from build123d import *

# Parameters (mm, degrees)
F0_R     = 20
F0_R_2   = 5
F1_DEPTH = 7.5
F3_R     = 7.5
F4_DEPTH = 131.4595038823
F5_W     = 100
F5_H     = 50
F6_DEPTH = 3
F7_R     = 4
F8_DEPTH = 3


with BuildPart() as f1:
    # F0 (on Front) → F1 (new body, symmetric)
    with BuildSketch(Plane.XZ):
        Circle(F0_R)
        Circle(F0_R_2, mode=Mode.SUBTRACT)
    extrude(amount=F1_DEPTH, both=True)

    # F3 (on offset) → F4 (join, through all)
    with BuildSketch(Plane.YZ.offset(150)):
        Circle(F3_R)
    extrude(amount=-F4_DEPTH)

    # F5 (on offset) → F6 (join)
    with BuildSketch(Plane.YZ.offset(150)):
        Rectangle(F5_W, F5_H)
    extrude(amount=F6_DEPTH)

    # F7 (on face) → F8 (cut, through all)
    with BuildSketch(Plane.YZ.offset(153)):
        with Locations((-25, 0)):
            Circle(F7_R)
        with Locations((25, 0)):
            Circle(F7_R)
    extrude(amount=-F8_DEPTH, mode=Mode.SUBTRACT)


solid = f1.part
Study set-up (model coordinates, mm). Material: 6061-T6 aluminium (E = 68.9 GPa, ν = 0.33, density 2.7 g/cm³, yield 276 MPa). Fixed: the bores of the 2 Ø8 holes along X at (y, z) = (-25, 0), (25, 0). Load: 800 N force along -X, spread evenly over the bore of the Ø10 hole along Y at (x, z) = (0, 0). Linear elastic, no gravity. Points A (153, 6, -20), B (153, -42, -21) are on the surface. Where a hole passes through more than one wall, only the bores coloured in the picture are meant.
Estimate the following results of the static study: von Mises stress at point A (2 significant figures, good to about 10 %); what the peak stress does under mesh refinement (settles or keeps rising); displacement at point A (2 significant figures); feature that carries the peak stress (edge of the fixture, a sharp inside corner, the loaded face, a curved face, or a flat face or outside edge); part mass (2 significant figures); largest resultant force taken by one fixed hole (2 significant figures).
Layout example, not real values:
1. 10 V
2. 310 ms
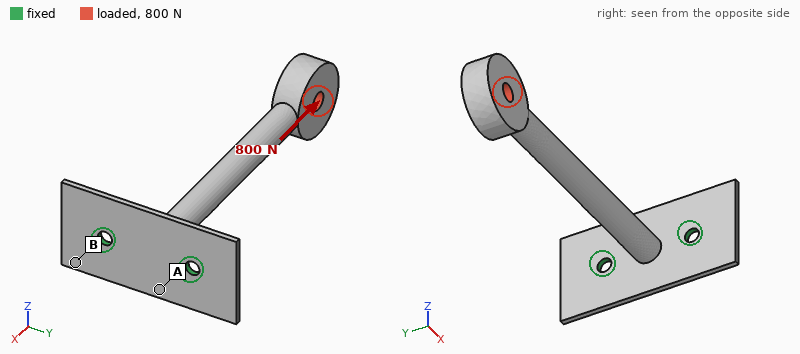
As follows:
1. 17 MPa
2. keeps rising
3. 40 µm
4. edge of the fixture
5. 150 g
6. 410 N
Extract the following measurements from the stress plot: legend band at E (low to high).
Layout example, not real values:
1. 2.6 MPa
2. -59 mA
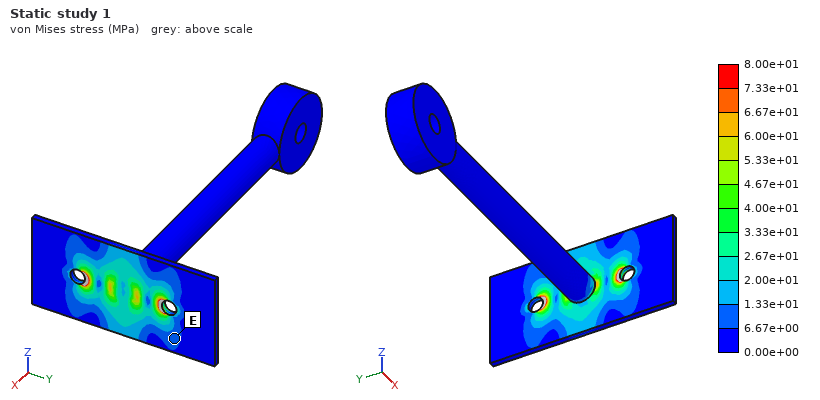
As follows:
1. 6.67e+00 to 1.33e+01 MPa
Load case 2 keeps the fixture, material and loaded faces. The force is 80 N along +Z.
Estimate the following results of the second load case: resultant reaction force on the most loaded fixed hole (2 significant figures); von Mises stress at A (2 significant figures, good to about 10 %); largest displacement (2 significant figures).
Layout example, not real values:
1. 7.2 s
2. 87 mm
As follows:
1. 40 N
2. 36 MPa
3. 2.2 mm
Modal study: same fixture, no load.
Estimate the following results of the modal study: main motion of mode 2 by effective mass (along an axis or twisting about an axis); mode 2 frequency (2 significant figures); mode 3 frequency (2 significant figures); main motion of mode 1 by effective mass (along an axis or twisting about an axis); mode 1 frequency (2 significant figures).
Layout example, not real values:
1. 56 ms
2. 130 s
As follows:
1. along Y
2. 180 Hz
3. 1400 Hz
4. along Z
5. 130 Hz
